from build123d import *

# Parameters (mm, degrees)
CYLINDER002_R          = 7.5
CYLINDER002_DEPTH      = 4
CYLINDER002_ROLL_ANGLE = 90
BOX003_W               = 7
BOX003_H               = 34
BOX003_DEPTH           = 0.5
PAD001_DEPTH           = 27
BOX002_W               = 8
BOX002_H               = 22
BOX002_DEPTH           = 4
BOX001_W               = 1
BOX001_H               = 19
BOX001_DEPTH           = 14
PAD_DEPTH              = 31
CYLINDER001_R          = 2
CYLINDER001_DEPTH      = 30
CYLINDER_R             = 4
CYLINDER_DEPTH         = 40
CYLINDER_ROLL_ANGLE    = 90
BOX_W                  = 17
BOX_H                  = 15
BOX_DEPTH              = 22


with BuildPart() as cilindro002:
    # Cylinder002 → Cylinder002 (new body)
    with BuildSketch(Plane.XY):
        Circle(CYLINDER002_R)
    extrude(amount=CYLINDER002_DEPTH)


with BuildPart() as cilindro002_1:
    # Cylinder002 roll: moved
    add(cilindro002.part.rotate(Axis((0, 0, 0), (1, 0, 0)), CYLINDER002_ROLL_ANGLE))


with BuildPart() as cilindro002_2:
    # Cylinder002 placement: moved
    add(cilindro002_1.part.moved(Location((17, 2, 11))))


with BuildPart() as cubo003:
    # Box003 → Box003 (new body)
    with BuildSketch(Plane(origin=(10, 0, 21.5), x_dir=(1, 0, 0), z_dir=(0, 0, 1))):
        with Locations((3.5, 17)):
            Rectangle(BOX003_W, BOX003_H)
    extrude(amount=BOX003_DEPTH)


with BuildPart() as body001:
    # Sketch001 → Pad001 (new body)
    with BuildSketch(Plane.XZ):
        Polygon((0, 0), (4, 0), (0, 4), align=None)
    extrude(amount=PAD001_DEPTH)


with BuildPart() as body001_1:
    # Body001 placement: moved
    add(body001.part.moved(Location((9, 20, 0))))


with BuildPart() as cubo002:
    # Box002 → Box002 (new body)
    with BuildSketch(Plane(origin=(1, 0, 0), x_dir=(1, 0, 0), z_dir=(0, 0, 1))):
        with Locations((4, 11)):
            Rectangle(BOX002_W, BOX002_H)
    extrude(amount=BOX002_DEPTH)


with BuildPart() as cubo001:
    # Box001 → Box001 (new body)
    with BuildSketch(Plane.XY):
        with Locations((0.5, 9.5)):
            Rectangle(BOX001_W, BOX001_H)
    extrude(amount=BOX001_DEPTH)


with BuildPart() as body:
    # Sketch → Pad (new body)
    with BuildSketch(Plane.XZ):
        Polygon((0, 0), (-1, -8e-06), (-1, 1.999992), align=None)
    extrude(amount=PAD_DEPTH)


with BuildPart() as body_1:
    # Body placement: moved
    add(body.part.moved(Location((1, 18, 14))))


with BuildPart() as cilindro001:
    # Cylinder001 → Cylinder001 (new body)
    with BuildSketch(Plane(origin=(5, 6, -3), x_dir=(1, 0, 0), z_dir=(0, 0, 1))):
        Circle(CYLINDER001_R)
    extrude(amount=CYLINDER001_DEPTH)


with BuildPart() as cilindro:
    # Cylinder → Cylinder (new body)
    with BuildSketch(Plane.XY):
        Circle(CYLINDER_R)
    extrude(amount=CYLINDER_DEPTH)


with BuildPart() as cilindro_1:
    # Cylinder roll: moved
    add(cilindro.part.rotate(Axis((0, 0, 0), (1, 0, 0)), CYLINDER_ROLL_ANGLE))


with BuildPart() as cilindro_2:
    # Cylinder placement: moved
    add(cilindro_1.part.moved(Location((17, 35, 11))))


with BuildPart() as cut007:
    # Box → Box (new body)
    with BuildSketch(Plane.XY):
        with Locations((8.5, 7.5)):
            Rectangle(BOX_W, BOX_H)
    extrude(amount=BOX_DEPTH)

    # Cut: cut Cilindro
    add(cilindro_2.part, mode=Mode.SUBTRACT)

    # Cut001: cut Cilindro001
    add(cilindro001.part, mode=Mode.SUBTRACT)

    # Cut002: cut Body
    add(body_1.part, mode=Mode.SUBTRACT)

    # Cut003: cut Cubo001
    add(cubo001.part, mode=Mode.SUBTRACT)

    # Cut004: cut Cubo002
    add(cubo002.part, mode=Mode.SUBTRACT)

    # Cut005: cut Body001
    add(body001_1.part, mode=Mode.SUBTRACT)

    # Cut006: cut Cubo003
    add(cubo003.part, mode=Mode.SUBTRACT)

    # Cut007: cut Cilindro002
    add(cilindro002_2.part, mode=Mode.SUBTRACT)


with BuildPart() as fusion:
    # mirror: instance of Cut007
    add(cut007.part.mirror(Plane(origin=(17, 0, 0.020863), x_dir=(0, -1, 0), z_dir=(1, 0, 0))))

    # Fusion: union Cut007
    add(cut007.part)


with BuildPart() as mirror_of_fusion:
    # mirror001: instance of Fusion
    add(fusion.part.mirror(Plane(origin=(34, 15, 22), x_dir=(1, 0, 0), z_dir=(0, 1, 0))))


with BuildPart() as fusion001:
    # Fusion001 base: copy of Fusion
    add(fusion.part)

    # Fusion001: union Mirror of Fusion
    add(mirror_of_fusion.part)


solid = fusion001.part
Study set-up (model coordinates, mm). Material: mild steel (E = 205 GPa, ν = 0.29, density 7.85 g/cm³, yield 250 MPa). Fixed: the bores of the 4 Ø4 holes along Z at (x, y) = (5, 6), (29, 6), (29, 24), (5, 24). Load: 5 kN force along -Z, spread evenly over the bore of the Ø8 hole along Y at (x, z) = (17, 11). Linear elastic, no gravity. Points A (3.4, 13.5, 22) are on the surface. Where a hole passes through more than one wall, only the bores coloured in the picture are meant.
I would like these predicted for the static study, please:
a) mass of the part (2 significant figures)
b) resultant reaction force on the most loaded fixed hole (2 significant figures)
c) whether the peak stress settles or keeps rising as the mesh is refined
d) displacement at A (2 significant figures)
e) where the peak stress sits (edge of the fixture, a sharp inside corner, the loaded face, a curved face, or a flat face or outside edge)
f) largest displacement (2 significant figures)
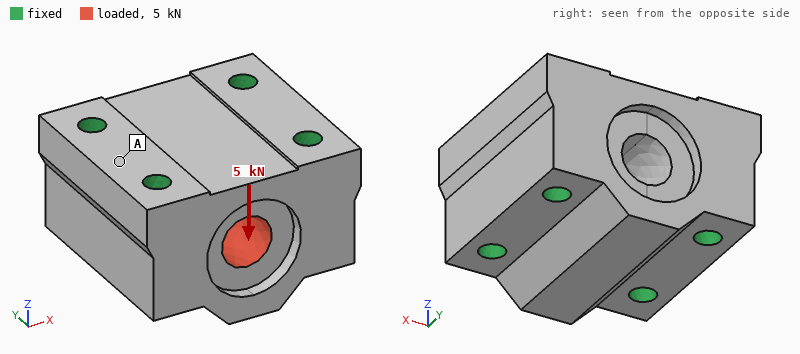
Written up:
130 g
2.0 kN
keeps rising
0.25 µm
edge of the fixture
1.5 µm
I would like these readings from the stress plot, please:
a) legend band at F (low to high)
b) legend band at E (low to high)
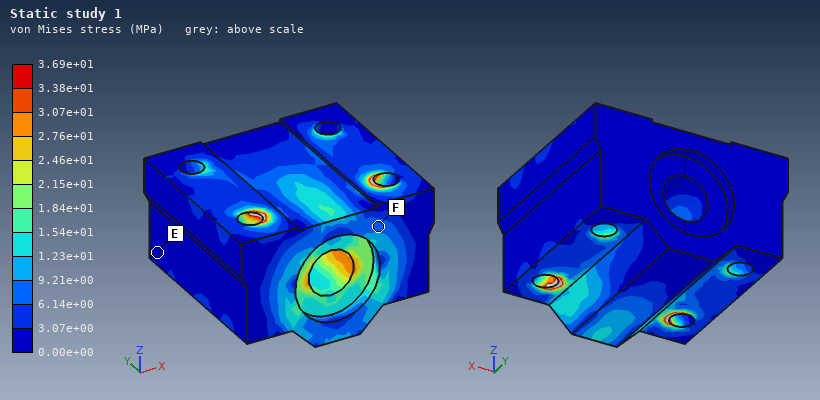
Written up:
6.14e+00 to 9.21e+00 MPa
0.00e+00 to 3.07e+00 MPa
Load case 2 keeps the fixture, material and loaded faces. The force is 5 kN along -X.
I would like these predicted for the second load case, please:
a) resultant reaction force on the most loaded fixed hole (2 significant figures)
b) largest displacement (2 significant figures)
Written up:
2.0 kN
0.76 µm
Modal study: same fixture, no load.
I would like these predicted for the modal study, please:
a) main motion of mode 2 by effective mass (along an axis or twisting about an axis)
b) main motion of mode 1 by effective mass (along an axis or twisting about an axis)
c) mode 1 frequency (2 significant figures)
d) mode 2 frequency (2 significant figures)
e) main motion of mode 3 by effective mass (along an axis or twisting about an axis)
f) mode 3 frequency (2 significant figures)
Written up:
along Z
along Y
54 kHz
59 kHz
along Y
67 kHz
